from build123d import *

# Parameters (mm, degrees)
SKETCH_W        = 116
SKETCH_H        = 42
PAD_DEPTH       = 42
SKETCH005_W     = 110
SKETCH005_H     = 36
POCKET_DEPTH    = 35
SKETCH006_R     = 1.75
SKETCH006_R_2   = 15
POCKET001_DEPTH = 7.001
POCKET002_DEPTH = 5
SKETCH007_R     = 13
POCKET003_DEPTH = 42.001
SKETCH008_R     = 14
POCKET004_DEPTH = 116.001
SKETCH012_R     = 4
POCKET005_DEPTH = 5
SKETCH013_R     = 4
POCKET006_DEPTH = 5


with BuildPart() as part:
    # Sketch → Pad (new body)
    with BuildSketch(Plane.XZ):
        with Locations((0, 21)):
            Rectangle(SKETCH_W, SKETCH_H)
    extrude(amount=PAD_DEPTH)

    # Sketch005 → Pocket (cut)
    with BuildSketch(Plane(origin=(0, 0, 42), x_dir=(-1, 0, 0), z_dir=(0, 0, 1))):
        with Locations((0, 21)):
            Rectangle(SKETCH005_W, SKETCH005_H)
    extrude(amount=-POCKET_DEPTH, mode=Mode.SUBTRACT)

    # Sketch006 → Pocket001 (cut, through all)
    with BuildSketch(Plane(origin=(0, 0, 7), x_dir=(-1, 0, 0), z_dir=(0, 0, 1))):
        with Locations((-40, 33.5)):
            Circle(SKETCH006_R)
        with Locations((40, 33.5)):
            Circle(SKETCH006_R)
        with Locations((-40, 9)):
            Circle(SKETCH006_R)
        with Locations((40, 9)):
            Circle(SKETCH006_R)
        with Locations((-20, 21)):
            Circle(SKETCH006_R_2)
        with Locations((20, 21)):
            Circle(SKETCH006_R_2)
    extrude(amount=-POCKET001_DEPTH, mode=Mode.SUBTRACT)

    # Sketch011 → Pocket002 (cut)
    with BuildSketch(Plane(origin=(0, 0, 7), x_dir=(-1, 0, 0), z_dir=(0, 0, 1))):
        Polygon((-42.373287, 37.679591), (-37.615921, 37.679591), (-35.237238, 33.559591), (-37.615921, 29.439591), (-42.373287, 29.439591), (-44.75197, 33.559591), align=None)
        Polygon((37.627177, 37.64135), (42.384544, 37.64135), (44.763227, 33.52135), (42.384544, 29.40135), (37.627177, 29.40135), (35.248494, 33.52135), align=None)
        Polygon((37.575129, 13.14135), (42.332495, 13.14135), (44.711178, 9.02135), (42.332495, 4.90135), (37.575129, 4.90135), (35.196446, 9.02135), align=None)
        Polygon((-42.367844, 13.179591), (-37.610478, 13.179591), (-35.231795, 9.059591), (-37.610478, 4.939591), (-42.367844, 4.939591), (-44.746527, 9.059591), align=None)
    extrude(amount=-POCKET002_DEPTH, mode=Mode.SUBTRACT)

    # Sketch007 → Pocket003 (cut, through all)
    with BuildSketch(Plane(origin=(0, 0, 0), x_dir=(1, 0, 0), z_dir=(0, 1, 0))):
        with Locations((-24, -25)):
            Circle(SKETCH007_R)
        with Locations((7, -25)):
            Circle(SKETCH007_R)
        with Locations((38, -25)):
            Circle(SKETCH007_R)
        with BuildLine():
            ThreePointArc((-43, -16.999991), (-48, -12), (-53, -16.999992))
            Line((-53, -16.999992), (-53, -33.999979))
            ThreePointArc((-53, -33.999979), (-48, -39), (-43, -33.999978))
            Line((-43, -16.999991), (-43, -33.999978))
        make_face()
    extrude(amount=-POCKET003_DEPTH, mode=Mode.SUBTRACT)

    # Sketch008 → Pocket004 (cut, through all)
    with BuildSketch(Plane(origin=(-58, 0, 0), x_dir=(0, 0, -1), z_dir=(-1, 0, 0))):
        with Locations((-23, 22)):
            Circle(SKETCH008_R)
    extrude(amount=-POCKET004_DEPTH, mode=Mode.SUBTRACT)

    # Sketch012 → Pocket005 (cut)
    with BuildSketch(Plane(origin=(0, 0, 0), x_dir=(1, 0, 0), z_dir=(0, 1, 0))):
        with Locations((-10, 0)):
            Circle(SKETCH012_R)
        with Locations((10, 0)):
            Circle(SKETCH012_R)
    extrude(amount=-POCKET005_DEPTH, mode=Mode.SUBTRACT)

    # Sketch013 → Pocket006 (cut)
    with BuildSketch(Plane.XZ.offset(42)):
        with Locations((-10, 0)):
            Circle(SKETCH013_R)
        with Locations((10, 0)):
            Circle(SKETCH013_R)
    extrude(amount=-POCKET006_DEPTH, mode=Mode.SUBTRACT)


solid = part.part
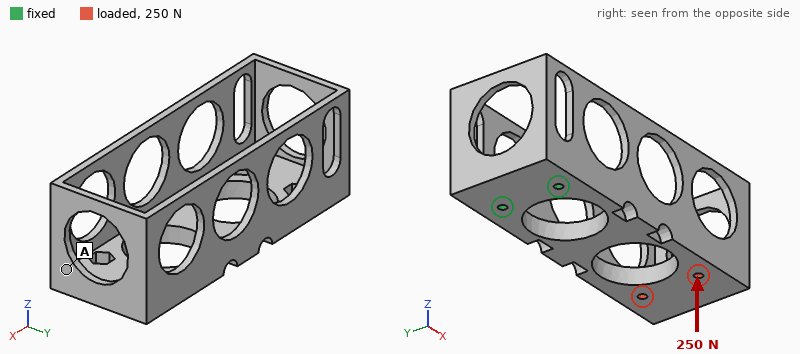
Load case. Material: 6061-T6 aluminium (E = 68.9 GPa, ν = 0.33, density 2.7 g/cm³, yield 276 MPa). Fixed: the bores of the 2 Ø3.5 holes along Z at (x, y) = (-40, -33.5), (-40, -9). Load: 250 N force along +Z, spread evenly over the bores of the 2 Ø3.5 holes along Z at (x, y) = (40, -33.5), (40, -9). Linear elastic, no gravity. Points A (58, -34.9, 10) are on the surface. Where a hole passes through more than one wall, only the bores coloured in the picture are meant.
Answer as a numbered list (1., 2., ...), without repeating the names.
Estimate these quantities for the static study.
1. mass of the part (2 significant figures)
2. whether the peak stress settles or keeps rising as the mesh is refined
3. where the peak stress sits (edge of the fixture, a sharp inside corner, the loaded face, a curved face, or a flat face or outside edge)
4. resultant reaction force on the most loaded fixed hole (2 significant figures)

1. 110 g
2. keeps rising
3. edge of the fixture
4. 270 N
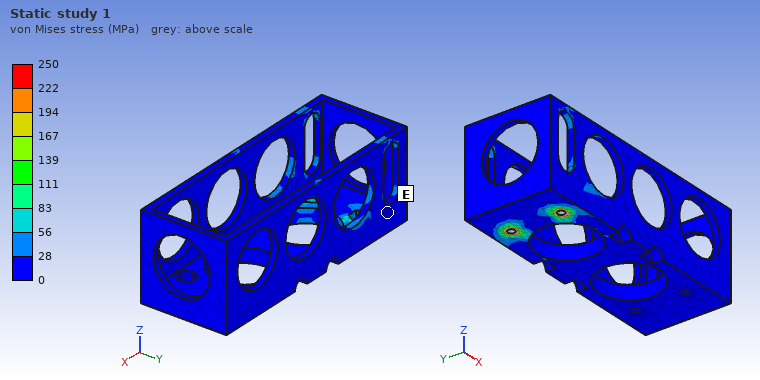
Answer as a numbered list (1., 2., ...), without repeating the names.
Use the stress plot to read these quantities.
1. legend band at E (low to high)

1. 0 to 28 MPa
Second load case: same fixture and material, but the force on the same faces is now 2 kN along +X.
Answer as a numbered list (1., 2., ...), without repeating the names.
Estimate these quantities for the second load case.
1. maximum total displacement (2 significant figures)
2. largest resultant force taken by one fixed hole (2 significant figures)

1. 93 µm
2. 1.0 kN
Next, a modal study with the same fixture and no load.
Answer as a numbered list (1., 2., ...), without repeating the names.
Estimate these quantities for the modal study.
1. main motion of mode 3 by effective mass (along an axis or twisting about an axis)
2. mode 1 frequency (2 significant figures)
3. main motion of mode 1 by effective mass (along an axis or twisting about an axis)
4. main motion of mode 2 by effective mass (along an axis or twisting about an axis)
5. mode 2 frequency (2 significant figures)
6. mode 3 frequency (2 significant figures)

1. along Y
2. 330 Hz
3. along Z
4. along Y
5. 940 Hz
6. 1500 Hz
